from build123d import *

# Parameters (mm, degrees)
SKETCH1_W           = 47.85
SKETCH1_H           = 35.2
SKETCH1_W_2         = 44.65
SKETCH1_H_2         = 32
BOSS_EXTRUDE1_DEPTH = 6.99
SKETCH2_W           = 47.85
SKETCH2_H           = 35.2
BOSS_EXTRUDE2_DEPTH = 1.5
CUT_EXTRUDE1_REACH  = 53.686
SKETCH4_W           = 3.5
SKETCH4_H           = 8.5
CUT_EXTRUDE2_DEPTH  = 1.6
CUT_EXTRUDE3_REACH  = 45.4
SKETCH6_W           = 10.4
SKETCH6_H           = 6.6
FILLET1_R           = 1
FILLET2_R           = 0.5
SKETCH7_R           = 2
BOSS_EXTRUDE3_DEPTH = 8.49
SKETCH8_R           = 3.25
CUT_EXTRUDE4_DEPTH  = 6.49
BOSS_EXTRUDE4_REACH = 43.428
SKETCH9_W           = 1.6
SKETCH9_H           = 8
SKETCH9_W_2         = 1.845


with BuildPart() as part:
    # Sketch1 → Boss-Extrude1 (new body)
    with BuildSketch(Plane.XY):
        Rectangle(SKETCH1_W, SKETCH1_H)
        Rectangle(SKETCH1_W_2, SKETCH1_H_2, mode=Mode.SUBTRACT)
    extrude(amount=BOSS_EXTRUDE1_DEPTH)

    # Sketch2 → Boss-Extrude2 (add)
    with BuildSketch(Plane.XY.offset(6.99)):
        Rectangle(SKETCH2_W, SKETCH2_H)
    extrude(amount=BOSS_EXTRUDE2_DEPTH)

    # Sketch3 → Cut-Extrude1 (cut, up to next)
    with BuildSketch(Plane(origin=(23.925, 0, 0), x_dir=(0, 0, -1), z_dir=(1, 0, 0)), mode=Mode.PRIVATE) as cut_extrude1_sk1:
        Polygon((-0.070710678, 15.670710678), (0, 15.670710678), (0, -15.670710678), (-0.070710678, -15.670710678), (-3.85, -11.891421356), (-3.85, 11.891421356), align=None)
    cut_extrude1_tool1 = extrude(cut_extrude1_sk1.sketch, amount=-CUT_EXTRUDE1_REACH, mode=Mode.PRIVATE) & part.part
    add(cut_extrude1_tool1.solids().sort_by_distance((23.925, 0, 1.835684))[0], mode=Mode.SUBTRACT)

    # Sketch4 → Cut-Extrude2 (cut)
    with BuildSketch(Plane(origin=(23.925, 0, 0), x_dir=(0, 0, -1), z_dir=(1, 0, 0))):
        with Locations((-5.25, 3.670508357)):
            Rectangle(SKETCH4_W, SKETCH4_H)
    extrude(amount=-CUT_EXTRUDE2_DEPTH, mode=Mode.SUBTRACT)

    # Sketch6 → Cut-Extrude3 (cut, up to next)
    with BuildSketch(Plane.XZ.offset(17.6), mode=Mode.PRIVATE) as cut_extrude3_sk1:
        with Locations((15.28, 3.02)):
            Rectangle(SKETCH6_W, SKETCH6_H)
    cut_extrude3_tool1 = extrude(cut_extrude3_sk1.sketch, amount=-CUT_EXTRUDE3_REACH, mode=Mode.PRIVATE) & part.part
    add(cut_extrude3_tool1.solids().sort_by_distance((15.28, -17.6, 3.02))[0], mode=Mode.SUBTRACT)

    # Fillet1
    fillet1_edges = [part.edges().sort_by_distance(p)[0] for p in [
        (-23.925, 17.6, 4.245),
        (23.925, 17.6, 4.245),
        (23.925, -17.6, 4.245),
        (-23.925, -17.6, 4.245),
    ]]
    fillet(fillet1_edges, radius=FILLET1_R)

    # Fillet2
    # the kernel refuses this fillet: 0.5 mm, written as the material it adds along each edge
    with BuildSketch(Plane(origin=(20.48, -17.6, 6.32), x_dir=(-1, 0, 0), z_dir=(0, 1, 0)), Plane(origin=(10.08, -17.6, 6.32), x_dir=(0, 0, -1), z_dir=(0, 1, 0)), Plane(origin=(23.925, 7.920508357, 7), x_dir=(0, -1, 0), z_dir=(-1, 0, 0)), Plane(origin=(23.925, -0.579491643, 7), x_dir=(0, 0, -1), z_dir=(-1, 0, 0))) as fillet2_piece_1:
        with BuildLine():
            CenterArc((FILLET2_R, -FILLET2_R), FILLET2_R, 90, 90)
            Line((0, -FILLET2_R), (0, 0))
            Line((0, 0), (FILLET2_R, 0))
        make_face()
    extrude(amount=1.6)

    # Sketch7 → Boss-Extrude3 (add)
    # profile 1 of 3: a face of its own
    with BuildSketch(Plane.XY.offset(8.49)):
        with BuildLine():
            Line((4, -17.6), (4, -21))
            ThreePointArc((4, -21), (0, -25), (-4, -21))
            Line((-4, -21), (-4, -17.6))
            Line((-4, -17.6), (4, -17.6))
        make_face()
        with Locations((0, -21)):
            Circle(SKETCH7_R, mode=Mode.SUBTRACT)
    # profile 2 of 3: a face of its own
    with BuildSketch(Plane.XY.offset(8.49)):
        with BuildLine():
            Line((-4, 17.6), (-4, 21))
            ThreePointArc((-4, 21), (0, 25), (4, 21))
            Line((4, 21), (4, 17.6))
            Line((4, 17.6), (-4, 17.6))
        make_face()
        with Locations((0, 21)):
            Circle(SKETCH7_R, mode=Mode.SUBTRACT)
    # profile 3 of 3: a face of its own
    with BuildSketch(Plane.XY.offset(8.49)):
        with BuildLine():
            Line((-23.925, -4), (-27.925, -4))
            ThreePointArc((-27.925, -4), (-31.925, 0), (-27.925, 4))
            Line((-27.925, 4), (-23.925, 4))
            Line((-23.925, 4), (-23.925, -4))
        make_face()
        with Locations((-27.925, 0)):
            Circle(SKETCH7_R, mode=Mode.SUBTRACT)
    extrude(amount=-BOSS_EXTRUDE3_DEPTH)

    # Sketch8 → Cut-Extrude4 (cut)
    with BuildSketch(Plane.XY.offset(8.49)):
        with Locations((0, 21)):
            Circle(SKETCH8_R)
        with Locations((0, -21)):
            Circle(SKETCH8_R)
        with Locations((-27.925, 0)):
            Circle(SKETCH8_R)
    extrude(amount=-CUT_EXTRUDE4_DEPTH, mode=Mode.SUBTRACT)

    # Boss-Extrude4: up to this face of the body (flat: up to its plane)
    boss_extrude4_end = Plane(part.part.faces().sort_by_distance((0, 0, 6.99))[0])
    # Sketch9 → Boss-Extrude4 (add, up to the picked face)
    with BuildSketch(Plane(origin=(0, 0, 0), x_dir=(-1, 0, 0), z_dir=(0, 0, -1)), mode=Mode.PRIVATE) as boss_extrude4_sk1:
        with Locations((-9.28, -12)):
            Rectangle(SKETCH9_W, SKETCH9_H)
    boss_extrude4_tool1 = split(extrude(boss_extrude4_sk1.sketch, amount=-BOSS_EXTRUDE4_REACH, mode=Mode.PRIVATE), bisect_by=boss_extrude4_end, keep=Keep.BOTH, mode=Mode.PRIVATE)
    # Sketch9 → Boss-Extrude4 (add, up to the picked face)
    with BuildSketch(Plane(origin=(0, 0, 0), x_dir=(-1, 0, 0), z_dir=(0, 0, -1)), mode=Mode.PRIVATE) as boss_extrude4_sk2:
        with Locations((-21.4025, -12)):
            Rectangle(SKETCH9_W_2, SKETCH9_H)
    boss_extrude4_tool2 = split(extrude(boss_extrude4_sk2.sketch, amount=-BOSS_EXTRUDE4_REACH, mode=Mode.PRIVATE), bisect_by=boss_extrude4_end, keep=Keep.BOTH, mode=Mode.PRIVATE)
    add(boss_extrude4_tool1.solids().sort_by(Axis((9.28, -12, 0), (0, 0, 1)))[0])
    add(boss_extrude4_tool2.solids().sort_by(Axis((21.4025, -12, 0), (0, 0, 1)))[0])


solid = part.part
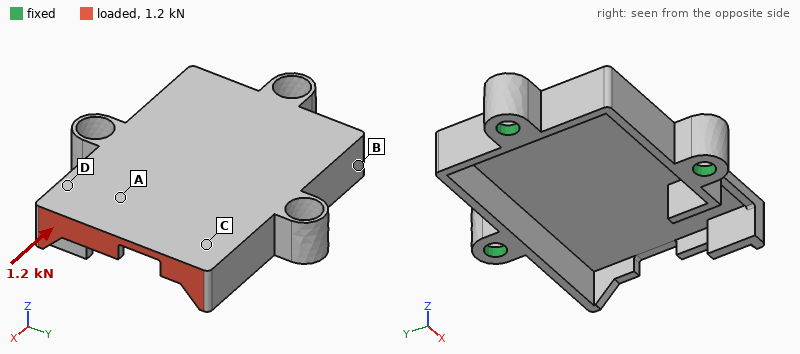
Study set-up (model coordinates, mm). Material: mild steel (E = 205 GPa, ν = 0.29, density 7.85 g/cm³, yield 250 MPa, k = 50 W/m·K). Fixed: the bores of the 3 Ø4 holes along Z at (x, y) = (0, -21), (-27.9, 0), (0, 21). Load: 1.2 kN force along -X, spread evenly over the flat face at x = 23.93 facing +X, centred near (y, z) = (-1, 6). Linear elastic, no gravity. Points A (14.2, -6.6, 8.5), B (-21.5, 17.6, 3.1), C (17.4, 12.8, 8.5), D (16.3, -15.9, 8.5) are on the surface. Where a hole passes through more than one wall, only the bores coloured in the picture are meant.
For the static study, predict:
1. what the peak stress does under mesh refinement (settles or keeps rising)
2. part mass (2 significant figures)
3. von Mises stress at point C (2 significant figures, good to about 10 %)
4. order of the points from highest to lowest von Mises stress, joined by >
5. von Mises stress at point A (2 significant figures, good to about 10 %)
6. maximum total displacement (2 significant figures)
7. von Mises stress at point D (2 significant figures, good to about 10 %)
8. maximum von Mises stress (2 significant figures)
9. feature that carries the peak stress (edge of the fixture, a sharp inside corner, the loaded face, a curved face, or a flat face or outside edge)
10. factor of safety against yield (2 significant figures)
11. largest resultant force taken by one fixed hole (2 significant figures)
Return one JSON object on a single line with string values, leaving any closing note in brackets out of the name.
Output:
{"what the peak stress does under mesh refinement": "settles", "part mass": "38 g", "von Mises stress at point C": "29 MPa", "order of the points from highest to lowest von Mises stress, joined by >": "D > A > C > B", "von Mises stress at point A": "69 MPa", "maximum total displacement": "0.11 mm", "von Mises stress at point D": "130 MPa", "maximum von Mises stress": "420 MPa", "feature that carries the peak stress": "a curved face", "factor of safety against yield": "0.59", "largest resultant force taken by one fixed hole": "480 N"}
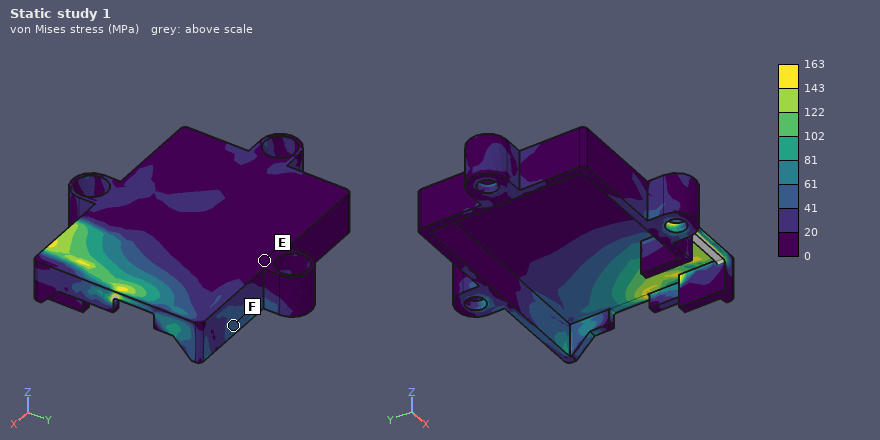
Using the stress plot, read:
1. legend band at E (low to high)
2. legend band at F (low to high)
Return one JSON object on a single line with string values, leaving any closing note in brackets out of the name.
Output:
{"legend band at E": "0 to 20 MPa", "legend band at F": "41 to 61 MPa"}
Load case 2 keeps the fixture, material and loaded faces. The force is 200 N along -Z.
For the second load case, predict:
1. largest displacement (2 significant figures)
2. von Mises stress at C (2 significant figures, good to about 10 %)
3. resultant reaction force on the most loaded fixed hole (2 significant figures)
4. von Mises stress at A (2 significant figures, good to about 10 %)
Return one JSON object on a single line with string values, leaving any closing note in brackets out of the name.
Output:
{"largest displacement": "0.12 mm", "von Mises stress at C": "52 MPa", "resultant reaction force on the most loaded fixed hole": "220 N", "von Mises stress at A": "75 MPa"}
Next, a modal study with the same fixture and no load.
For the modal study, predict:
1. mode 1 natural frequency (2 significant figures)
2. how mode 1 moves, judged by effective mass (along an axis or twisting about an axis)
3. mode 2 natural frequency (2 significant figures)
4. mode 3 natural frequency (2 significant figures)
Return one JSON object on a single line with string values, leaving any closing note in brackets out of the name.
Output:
{"mode 1 natural frequency": "3400 Hz", "how mode 1 moves, judged by effective mass": "along Z", "mode 2 natural frequency": "5700 Hz", "mode 3 natural frequency": "7400 Hz"}
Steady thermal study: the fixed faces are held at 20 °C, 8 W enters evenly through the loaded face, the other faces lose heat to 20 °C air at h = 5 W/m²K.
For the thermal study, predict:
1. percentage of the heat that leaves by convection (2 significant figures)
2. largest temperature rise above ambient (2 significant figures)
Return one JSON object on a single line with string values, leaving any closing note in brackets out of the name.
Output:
{"percentage of the heat that leaves by convection": "8.6 %", "largest temperature rise above ambient": "75 K"}
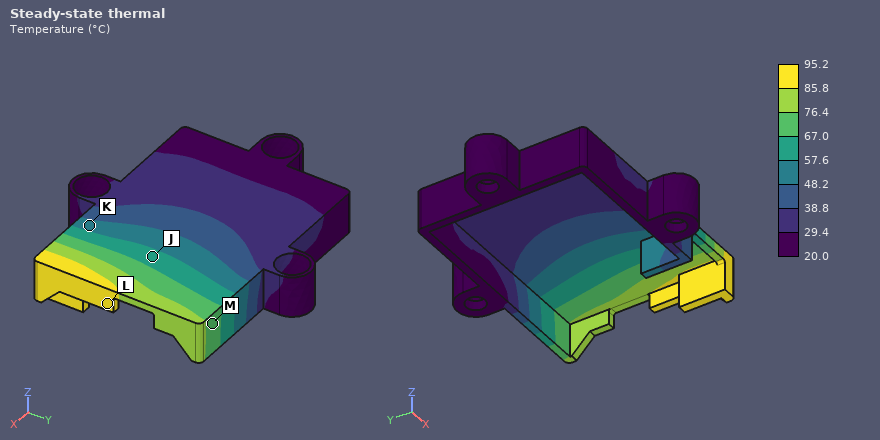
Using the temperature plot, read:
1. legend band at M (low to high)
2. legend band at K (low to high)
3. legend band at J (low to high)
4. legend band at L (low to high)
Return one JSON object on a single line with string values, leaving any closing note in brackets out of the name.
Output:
{"legend band at M": "67.0 to 76.4 °C", "legend band at K": "48.2 to 57.6 °C", "legend band at J": "57.6 to 67.0 °C", "legend band at L": "85.8 to 95.2 °C"}
